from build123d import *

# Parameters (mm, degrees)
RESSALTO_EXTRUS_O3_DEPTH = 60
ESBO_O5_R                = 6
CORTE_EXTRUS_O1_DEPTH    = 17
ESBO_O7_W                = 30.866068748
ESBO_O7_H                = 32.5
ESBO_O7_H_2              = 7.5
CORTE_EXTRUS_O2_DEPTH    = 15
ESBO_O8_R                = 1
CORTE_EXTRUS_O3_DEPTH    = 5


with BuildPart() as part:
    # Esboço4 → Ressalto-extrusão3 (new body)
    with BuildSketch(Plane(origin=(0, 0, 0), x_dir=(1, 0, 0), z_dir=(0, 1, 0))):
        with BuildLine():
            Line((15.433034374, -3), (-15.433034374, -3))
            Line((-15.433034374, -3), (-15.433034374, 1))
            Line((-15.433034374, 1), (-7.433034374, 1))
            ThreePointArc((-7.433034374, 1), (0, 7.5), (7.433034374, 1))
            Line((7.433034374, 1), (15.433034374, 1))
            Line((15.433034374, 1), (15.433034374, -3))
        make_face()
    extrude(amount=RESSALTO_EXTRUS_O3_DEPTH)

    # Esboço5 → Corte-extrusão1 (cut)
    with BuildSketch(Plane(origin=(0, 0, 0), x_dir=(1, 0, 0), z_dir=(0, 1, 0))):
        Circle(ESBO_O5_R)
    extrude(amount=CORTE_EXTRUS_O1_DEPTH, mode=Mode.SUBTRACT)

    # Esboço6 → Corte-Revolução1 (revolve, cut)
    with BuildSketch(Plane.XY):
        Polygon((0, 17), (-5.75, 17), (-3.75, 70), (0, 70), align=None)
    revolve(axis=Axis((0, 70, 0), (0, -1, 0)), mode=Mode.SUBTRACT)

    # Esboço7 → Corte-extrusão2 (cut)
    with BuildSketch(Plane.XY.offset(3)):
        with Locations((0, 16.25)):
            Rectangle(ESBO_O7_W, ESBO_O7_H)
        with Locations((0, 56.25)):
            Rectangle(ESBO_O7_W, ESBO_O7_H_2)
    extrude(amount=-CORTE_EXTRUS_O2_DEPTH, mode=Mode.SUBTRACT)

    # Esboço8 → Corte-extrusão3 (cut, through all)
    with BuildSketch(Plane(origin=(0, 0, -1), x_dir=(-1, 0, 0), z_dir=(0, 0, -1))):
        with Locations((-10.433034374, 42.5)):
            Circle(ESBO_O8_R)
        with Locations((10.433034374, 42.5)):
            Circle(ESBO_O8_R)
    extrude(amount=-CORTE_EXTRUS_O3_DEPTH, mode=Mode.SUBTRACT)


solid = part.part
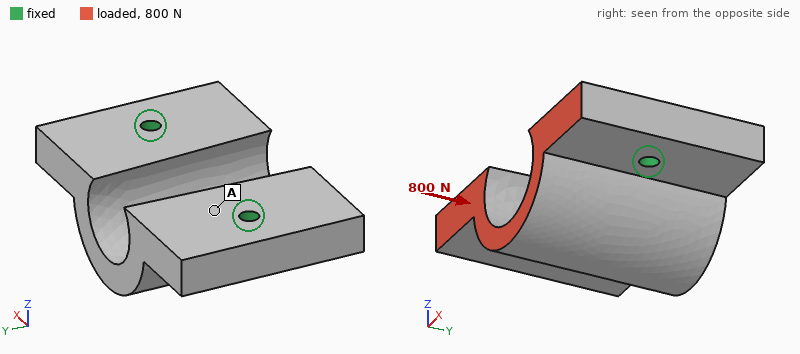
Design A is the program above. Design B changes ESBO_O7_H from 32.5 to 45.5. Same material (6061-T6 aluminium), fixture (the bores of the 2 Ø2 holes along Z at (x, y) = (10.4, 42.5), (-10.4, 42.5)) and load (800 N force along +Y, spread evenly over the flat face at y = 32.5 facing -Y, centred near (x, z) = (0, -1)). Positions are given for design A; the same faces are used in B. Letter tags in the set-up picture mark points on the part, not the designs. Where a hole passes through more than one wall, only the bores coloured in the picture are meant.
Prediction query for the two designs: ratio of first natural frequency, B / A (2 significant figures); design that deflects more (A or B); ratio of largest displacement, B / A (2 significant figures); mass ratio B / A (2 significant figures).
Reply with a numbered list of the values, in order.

1. 1.1
2. B
3. 1.2
4. 0.69
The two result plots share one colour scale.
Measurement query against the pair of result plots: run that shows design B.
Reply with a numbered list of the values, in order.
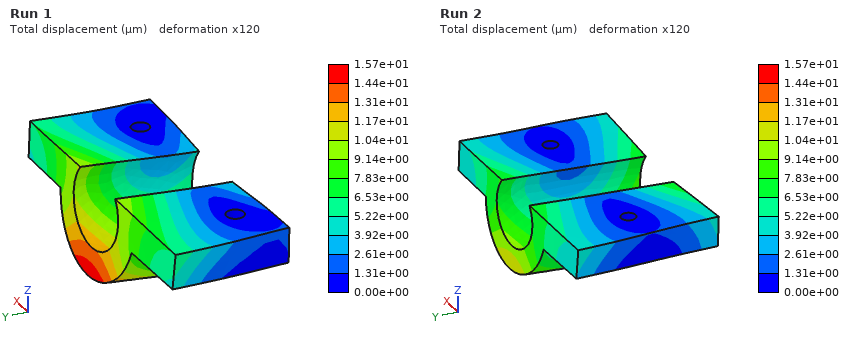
1. Run 1
